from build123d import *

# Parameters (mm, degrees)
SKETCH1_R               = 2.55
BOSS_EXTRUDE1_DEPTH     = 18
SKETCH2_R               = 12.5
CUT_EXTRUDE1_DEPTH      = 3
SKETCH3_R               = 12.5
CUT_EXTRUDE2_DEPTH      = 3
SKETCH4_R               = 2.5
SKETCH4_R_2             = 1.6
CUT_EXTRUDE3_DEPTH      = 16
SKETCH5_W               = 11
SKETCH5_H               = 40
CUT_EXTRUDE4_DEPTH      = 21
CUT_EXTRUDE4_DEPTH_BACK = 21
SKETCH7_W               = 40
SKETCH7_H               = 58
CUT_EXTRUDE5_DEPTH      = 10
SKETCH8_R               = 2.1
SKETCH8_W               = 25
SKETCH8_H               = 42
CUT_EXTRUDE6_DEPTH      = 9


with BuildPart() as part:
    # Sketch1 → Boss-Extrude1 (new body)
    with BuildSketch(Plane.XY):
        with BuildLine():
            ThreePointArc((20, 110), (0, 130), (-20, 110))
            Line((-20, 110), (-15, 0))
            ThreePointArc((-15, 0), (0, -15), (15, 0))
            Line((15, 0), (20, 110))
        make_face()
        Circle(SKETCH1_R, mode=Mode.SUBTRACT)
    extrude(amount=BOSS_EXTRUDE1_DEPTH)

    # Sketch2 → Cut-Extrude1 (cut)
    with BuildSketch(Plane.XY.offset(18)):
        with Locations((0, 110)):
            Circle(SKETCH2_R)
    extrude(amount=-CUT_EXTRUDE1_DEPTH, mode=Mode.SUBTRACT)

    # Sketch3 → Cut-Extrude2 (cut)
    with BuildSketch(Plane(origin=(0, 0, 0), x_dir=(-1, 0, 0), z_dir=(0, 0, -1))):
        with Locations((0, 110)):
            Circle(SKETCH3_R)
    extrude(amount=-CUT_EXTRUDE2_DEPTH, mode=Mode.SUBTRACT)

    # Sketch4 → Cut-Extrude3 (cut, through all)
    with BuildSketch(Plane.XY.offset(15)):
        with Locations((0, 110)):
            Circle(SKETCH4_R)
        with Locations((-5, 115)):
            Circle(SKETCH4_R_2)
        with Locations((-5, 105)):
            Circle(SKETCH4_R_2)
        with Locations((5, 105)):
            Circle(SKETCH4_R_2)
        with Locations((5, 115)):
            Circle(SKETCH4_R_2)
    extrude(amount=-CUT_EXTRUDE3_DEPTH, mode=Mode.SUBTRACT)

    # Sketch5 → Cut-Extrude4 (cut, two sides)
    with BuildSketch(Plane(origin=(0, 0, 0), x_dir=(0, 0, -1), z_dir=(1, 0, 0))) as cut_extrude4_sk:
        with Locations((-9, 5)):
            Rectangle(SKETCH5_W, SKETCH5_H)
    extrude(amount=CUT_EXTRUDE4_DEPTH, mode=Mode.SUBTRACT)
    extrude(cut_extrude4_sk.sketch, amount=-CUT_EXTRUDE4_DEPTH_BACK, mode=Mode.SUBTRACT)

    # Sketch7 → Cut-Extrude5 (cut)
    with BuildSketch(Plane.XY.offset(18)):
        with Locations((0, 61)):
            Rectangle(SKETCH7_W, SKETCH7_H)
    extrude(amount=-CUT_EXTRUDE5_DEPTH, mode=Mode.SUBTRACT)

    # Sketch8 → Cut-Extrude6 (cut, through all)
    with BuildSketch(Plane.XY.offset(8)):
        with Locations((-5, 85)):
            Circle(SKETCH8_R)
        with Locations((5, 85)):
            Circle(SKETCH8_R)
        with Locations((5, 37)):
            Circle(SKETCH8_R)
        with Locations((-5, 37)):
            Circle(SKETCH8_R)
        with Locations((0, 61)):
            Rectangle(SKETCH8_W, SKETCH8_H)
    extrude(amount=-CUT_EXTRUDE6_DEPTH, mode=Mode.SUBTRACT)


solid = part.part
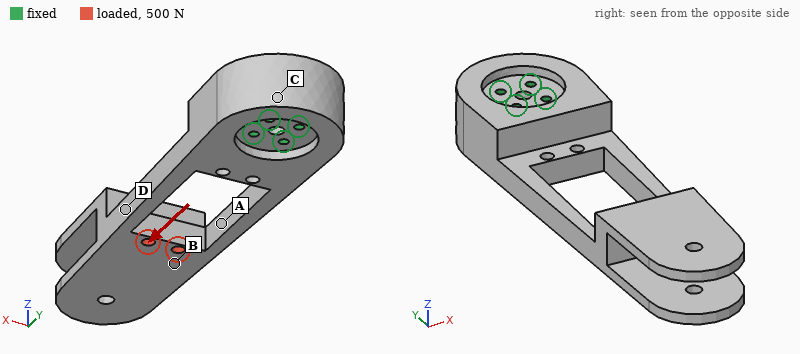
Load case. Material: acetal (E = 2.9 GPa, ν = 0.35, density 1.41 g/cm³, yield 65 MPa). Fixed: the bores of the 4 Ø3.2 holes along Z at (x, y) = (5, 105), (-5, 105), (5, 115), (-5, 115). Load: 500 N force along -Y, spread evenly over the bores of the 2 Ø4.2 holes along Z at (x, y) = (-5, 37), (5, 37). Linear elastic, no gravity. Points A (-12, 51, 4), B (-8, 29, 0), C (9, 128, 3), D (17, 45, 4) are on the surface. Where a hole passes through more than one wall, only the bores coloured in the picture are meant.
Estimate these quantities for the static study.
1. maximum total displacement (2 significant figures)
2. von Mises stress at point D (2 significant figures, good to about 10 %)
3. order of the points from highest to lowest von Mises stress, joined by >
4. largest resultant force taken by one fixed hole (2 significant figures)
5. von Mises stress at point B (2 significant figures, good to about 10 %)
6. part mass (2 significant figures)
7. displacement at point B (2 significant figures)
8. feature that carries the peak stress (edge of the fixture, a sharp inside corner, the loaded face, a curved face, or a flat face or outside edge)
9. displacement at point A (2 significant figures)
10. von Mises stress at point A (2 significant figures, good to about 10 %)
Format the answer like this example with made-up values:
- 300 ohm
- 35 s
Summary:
- 0.23 mm
- 5.0 MPa
- A > D > B > C
- 170 N
- 3.6 MPa
- 58 g
- 0.19 mm
- a flat face or outside edge
- 0.13 mm
- 8.2 MPa
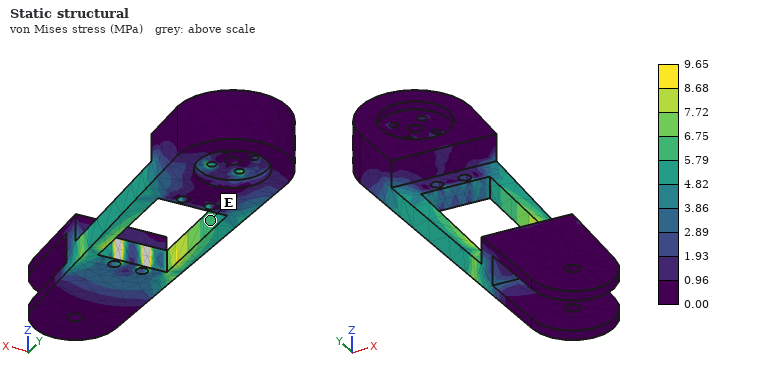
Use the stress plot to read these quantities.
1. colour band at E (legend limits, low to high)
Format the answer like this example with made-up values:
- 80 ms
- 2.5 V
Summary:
- 5.79 to 6.75 MPa
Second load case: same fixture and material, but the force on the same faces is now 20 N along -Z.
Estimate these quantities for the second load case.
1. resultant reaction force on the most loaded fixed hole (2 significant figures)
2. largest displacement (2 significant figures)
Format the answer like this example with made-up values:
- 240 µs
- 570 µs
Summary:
- 28 N
- 1.8 mm
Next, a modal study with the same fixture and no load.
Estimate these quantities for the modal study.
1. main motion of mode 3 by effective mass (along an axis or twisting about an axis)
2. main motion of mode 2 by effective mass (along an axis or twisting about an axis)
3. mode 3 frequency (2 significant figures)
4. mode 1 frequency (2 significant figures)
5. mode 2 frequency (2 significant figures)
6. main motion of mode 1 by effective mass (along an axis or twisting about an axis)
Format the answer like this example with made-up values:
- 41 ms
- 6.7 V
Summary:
- twisting about Y
- along X
- 500 Hz
- 110 Hz
- 250 Hz
- along Z
